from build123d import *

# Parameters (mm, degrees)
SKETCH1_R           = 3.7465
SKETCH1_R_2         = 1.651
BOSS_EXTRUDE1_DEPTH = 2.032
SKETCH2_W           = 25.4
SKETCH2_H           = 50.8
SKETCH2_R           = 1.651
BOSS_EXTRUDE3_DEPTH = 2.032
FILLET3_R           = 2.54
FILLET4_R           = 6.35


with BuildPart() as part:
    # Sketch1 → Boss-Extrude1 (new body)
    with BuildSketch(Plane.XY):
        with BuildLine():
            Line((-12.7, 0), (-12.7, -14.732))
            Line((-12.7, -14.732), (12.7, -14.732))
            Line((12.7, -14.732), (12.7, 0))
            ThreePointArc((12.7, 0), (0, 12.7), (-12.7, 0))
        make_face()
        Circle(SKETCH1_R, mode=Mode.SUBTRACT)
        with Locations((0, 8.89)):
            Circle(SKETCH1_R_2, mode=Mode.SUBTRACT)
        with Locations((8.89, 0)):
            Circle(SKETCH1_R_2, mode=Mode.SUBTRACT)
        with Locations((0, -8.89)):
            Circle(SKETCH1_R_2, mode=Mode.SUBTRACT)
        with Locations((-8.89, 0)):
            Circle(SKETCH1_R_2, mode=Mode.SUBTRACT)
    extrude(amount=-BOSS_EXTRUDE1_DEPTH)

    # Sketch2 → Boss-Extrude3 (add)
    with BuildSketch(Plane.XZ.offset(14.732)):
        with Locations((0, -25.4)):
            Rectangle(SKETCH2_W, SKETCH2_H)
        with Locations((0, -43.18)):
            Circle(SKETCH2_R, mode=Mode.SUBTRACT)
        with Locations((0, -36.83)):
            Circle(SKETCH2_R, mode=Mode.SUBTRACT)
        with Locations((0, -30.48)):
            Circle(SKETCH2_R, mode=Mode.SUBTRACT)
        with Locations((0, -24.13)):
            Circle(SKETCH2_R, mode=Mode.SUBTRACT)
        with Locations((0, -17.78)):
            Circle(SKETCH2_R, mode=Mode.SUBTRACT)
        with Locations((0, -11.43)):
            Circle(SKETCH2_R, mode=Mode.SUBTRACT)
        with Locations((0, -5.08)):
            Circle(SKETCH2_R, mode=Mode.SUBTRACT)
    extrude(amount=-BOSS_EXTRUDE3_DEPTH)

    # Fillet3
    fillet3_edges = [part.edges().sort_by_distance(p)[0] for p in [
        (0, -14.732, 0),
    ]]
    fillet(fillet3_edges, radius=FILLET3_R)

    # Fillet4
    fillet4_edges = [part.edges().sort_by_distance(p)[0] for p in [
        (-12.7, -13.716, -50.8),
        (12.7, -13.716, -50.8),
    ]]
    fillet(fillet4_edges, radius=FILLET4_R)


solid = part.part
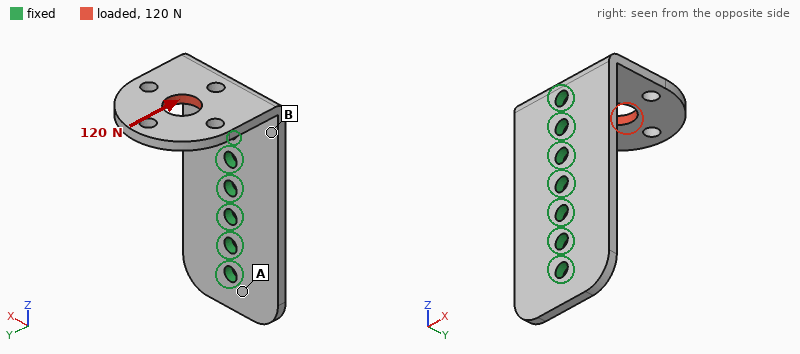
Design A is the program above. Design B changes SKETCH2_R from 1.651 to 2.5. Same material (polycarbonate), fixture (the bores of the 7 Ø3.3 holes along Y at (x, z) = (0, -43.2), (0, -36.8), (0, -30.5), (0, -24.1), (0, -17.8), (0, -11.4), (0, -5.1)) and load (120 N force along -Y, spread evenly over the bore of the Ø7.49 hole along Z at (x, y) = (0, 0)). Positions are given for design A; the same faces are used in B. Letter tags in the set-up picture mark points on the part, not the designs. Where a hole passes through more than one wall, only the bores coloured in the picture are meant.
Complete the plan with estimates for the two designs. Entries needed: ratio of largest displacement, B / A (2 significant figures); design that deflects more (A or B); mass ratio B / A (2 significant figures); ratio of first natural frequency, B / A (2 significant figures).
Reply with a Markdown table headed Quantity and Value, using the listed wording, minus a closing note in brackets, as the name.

| Quantity | Value |
|---|---|
| ratio of largest displacement, B / A | 0.61 |
| design that deflects more | A |
| mass ratio B / A | 0.95 |
| ratio of first natural frequency, B / A | 1.1 |
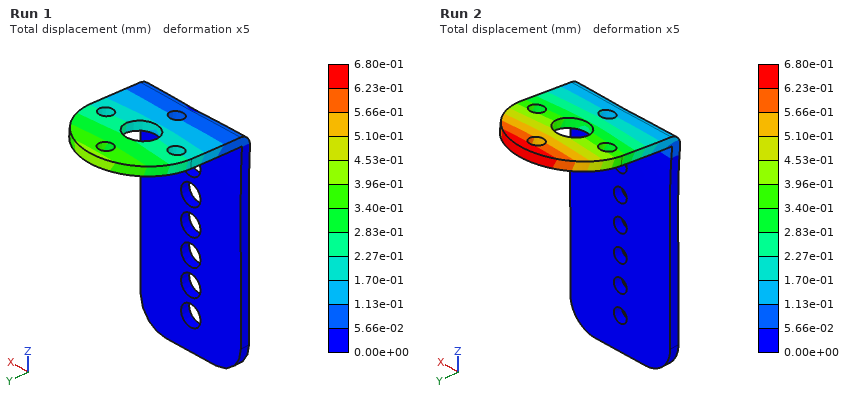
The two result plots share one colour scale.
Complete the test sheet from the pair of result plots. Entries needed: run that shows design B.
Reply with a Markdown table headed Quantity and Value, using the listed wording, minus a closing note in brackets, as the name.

| Quantity | Value |
|---|---|
| run that shows design B | Run 1 |
